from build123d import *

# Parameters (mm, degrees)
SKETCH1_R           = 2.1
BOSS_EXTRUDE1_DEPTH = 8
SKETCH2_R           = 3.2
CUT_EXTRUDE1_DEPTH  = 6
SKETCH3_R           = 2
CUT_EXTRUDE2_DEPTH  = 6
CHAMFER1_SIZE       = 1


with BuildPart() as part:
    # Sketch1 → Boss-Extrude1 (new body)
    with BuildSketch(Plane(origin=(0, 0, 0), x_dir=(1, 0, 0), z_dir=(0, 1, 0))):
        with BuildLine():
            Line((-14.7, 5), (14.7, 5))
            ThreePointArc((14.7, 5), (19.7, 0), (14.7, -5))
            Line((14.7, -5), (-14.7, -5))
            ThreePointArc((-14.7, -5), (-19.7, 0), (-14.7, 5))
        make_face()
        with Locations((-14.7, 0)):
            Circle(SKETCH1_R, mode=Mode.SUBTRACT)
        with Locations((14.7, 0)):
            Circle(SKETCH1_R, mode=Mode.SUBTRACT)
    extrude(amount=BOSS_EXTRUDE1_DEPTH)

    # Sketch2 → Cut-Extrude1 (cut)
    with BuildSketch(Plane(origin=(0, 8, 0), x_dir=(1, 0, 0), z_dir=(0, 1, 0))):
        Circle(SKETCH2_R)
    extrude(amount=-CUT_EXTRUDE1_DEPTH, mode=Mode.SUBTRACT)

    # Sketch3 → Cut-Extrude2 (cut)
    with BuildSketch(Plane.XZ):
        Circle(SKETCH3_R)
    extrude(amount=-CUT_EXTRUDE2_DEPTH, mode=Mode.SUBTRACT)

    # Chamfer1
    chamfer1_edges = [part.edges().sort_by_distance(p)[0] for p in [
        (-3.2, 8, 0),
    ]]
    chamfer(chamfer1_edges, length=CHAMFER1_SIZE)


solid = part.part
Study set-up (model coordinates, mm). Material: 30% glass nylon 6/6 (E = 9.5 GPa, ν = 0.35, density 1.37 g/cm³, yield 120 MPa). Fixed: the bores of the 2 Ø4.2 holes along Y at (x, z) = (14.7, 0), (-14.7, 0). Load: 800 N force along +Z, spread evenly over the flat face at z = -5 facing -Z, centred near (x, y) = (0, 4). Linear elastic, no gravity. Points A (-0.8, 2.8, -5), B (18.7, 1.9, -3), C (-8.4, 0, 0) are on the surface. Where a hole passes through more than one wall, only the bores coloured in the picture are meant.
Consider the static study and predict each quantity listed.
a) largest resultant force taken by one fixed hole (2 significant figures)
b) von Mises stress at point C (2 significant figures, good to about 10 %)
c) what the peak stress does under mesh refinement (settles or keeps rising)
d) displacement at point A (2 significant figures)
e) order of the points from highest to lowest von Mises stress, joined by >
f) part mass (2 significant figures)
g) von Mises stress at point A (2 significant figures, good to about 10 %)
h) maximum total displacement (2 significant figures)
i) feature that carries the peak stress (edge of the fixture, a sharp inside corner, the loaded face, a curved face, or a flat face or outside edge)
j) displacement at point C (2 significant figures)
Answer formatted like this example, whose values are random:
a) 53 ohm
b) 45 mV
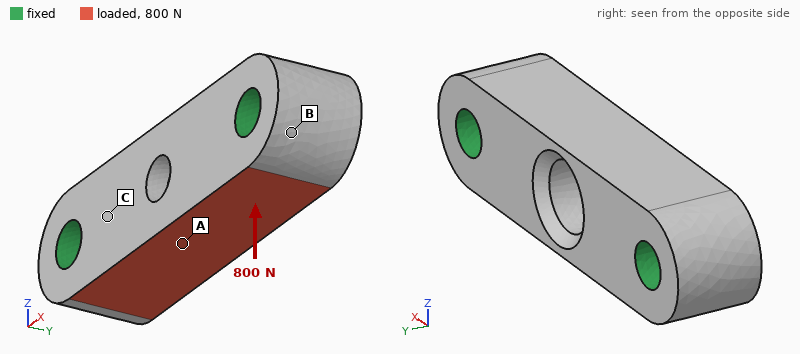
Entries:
a) 400 N
b) 7.9 MPa
c) keeps rising
d) 24 µm
e) A > C > B
f) 3.5 g
g) 13 MPa
h) 28 µm
i) edge of the fixture
j) 12 µm
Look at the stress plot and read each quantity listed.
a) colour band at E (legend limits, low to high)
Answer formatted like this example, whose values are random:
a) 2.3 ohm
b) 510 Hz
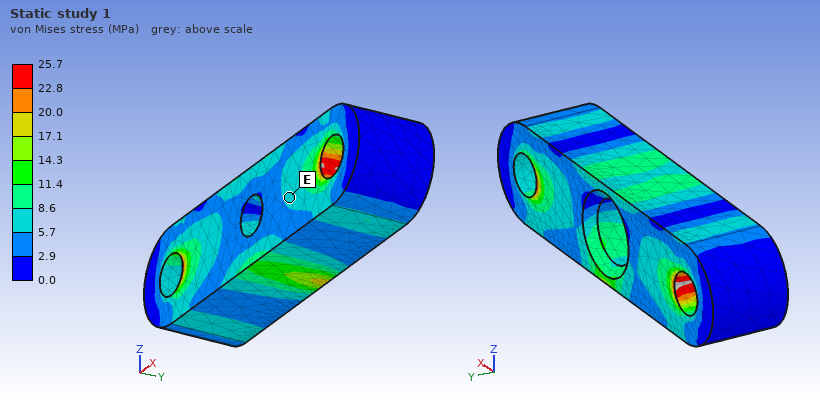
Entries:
a) 5.7 to 8.6 MPa
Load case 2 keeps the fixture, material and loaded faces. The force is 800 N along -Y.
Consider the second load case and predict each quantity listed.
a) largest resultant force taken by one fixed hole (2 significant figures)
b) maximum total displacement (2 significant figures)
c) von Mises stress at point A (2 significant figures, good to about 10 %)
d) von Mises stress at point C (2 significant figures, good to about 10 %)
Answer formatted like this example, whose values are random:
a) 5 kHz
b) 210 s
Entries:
a) 400 N
b) 58 µm
c) 8.1 MPa
d) 13 MPa
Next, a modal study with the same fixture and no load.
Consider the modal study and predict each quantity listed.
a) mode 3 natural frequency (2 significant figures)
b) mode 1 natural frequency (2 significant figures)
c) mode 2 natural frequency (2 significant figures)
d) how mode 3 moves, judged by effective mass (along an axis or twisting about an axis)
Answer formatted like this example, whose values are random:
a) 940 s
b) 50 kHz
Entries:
a) 28 kHz
b) 21 kHz
c) 21 kHz
d) twisting about X
